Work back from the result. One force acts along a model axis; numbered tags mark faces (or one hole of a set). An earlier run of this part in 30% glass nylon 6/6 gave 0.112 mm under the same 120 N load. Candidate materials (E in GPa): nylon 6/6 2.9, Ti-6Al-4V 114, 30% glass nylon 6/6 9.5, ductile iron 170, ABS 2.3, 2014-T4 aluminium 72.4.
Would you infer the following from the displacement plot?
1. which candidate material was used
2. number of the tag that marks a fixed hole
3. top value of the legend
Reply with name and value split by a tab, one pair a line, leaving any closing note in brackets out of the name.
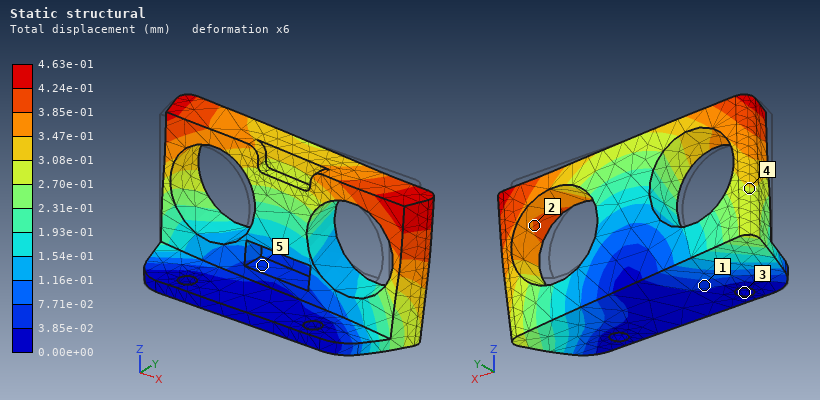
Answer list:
which candidate material was used	ABS
number of the tag that marks a fixed hole	3
top value of the legend	4.63e-01 mm
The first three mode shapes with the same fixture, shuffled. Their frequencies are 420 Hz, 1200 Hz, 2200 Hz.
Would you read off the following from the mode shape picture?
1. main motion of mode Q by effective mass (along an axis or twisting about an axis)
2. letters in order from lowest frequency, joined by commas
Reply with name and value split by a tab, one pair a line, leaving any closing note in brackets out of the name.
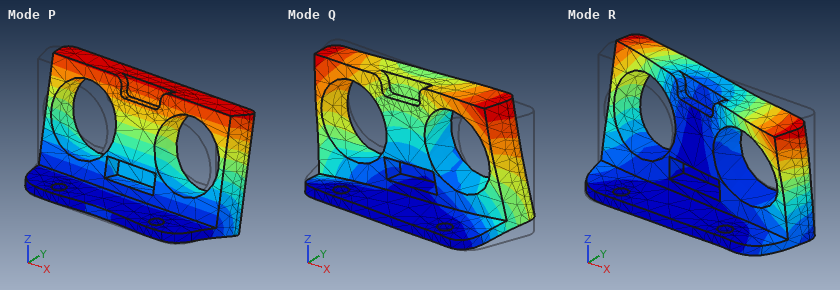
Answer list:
main motion of mode Q by effective mass	along X
letters in order from lowest frequency, joined by commas	P, Q, R
